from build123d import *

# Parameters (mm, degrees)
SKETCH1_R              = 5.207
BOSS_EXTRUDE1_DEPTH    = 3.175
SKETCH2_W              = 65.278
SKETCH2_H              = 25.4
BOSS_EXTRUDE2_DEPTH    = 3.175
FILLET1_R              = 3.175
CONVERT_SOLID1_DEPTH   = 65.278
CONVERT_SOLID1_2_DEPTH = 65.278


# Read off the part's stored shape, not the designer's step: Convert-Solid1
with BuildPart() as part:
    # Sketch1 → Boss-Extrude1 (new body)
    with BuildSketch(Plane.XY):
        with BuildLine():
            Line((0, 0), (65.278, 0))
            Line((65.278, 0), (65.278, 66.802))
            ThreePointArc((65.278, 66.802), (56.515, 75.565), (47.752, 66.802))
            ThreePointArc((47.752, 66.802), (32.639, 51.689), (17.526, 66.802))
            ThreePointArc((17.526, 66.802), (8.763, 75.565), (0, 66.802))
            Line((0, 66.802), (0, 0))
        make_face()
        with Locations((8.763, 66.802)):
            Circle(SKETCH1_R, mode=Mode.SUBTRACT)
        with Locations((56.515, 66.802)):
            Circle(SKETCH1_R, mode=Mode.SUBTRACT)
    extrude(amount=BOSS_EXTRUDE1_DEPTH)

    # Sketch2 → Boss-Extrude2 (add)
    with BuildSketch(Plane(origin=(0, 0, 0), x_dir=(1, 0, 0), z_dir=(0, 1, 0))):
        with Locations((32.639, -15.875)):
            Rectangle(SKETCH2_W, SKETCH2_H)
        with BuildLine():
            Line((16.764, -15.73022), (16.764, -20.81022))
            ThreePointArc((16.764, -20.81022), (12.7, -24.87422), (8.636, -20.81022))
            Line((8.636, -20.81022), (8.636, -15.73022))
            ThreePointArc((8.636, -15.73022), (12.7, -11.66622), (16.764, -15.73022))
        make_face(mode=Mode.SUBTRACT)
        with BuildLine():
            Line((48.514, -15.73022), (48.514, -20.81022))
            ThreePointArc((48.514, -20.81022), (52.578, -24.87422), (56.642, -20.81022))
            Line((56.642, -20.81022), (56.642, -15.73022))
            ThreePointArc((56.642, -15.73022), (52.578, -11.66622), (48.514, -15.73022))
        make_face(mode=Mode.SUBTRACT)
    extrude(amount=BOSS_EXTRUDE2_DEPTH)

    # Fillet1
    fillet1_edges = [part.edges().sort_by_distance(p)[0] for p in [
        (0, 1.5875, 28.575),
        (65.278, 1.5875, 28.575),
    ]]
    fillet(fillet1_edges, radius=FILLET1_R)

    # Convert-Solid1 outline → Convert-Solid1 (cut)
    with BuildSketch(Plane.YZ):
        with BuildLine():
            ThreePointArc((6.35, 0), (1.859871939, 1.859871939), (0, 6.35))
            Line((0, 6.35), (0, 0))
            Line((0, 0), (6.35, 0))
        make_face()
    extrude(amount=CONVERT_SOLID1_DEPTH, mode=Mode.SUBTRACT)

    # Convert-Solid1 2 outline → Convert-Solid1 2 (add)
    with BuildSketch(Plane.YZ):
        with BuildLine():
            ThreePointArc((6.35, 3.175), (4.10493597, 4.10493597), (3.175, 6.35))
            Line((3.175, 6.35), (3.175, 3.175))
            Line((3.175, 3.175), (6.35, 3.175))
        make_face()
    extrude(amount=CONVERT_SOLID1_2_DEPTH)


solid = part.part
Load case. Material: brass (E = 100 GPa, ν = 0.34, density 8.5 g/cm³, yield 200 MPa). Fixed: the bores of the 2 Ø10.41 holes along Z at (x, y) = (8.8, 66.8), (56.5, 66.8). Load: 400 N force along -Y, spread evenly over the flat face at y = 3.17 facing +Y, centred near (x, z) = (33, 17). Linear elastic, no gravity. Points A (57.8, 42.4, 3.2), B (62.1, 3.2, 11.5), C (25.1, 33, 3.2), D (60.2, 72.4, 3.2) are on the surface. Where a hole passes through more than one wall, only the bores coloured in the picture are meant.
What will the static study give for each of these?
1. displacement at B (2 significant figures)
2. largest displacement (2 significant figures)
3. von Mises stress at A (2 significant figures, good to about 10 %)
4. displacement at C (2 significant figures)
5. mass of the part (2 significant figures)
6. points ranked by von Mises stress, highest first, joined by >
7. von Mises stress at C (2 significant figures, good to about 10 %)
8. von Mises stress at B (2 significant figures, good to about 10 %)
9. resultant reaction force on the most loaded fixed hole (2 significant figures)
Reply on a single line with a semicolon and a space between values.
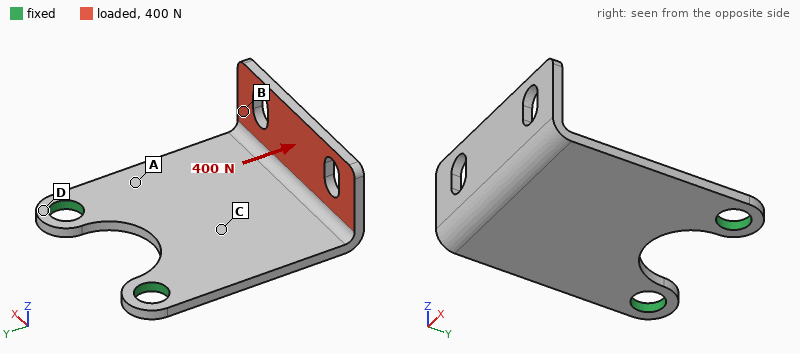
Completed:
0.81 mm; 1.1 mm; 65 MPa; 0.23 mm; 150 g; A > C > B > D; 52 MPa; 22 MPa; 210 N
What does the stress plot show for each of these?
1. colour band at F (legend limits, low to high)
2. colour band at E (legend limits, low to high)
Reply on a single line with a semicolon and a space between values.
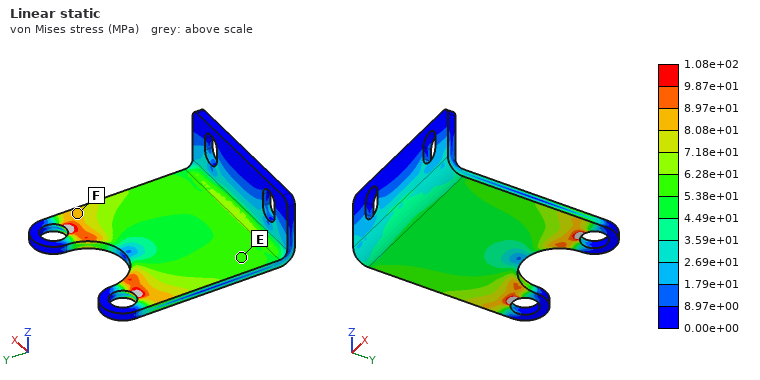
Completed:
8.08e+01 to 8.97e+01 MPa; 5.38e+01 to 6.28e+01 MPa
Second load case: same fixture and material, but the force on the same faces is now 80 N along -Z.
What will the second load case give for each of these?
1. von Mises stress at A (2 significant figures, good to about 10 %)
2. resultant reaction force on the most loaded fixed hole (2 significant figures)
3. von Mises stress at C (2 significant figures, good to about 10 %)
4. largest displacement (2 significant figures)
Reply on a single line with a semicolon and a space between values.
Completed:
32 MPa; 40 N; 19 MPa; 0.52 mm
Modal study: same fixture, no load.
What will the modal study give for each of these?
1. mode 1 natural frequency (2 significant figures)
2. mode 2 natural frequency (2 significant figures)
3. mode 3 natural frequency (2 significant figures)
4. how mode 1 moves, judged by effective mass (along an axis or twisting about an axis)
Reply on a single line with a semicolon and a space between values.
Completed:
250 Hz; 670 Hz; 1300 Hz; along Z
